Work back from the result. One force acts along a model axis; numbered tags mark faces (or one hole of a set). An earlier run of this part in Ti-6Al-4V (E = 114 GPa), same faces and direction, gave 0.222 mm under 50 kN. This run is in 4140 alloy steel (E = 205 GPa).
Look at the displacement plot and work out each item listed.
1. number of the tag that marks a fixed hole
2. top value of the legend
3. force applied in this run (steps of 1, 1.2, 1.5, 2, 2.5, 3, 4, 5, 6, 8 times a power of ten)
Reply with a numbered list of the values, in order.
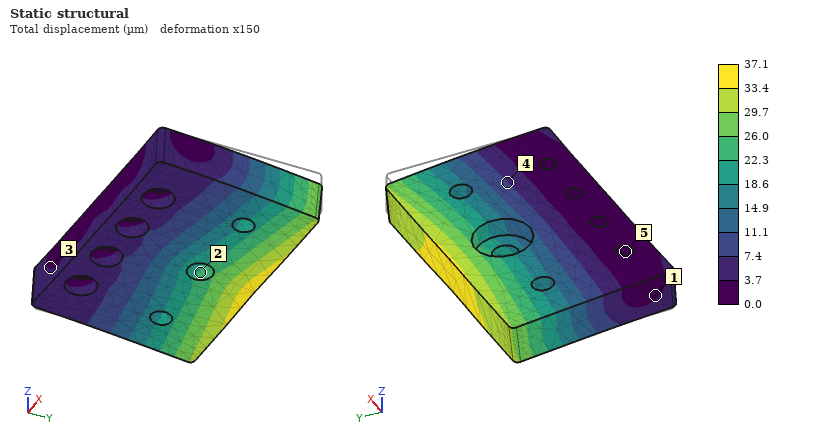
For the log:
1. 5
2. 37.1 µm
3. 15 kN
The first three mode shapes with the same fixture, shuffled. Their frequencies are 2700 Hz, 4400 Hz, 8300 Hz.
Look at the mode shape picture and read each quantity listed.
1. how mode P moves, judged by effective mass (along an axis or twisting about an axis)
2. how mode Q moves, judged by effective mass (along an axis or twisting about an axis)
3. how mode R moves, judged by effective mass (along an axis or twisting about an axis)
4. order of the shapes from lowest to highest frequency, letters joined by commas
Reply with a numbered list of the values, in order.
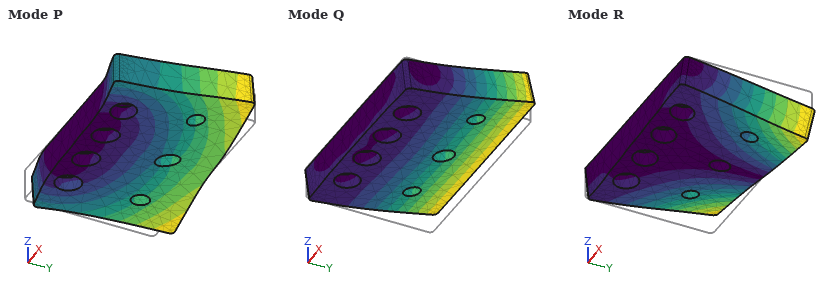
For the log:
1. along X
2. along Z
3. twisting about Y
4. Q, R, P
